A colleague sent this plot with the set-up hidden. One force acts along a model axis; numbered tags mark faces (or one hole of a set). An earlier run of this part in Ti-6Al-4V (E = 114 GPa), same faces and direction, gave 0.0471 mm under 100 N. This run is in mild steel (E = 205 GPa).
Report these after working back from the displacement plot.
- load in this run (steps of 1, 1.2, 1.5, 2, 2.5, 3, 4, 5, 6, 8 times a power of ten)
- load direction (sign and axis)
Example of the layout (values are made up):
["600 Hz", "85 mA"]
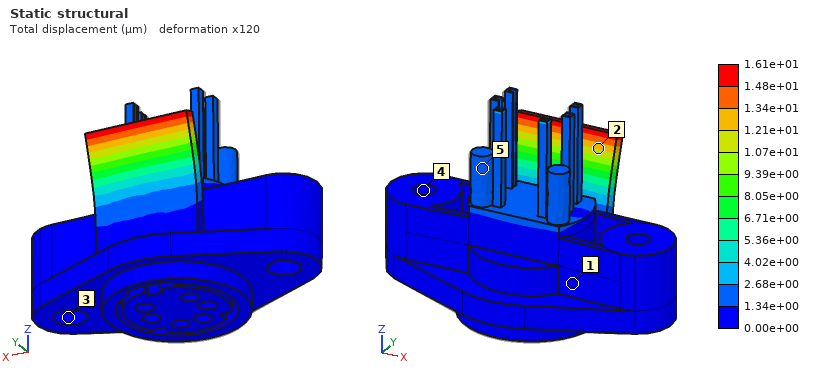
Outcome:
["60 N", "+Y"]
